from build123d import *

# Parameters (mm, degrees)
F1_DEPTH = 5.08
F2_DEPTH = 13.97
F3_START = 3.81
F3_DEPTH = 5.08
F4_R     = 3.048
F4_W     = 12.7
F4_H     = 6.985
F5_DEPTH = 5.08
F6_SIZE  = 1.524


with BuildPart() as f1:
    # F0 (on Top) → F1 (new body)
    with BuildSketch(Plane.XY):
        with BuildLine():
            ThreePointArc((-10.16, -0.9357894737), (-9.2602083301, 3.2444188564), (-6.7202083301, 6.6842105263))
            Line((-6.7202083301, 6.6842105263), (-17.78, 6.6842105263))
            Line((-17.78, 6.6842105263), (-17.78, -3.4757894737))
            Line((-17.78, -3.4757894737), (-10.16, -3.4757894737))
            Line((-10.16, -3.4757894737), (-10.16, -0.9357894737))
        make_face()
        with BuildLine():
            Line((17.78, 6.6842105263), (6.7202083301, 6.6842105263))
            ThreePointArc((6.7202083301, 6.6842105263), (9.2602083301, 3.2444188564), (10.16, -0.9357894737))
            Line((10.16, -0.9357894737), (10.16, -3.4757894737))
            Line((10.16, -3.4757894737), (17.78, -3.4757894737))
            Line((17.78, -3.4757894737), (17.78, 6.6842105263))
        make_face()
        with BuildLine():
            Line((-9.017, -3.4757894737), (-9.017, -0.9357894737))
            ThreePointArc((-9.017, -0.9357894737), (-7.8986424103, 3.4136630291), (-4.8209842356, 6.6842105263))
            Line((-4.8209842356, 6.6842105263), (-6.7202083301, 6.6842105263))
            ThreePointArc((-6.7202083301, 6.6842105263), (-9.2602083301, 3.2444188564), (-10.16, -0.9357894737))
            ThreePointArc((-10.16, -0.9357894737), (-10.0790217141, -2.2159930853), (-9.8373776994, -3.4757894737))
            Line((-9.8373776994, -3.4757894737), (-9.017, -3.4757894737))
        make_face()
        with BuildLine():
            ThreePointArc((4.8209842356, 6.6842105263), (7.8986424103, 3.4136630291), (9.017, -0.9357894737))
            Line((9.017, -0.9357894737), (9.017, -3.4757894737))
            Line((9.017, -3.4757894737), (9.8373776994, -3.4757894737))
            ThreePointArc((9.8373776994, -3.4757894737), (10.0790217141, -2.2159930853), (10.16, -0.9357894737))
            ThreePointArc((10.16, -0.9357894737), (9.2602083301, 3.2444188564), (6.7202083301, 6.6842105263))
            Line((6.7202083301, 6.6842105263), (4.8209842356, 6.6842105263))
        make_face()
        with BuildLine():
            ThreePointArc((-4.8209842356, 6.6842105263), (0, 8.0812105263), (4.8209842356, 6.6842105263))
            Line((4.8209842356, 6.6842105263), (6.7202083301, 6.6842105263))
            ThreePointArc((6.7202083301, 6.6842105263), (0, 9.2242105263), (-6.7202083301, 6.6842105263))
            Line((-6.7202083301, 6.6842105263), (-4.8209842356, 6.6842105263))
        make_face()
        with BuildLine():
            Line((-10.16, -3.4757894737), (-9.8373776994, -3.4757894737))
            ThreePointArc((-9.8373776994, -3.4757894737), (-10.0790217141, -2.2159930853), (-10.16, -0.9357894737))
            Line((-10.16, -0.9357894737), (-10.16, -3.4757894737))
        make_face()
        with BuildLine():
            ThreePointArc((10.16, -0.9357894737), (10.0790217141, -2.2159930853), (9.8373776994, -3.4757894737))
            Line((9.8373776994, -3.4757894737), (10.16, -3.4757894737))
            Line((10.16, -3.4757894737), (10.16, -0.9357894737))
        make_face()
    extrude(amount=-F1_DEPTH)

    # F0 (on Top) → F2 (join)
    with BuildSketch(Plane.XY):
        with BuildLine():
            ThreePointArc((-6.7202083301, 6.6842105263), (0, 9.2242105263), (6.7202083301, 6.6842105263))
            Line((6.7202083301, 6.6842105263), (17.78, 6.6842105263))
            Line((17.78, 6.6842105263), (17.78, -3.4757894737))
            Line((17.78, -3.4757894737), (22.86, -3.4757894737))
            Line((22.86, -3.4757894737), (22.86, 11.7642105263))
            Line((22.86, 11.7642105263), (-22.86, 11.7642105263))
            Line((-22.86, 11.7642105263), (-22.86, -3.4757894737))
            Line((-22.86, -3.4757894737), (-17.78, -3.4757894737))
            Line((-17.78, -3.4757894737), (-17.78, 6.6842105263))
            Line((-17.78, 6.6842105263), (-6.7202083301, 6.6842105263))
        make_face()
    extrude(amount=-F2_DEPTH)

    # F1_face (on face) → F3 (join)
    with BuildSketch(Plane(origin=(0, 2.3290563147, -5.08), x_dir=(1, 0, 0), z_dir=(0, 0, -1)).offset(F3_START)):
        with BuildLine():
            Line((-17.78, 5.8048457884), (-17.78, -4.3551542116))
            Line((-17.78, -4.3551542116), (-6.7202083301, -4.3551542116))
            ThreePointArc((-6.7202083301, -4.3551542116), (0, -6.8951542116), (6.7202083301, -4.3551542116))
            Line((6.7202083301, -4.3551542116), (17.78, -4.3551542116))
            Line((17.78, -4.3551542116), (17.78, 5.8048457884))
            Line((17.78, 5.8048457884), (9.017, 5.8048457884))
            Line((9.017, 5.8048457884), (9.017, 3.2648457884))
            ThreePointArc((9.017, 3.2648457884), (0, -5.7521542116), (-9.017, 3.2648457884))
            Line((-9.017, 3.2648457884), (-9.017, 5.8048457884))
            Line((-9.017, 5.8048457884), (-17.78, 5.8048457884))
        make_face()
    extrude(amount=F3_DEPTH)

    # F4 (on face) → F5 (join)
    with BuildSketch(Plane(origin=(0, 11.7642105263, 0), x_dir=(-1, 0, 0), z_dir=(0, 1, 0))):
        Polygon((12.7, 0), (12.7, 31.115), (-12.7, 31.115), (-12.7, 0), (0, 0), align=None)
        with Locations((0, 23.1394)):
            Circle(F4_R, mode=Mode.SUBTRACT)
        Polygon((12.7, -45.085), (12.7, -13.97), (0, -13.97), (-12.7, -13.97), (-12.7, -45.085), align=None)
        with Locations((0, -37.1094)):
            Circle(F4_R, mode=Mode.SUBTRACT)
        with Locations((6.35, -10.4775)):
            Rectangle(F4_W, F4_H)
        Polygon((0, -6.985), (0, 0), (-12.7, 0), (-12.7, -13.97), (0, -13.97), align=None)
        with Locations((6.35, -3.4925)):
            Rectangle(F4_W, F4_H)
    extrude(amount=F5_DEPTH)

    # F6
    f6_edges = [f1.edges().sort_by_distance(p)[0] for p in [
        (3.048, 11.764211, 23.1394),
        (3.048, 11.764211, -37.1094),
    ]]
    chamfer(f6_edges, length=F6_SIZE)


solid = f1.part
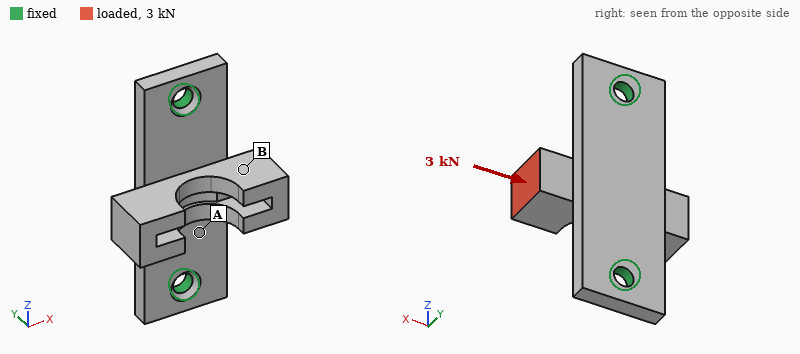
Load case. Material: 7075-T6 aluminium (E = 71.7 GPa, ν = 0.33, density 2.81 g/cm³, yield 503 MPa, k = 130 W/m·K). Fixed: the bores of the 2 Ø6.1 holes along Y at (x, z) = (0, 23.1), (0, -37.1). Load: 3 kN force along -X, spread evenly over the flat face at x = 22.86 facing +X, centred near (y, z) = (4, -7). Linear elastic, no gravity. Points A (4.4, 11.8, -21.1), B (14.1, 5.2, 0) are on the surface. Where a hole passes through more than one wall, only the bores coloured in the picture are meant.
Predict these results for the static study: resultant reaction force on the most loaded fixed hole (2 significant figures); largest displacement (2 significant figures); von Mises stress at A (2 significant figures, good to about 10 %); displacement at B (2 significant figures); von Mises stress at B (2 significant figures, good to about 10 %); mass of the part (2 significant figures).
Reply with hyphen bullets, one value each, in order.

- 1.5 kN
- 0.46 mm
- 140 MPa
- 0.26 mm
- 41 MPa
- 45 g
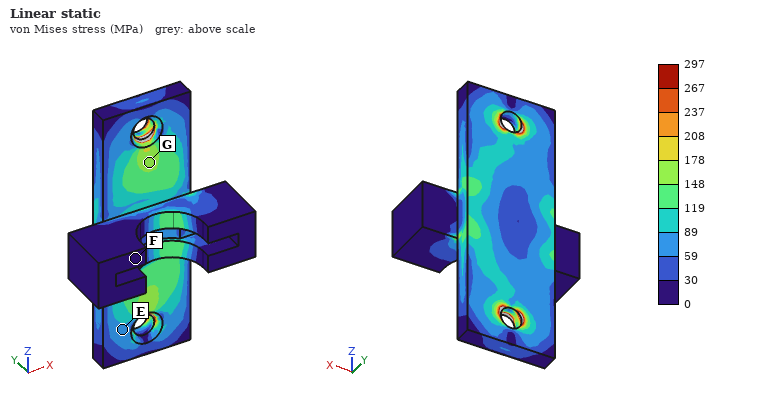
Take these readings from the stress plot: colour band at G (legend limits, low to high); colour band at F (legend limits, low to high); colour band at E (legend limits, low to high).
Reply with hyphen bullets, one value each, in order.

- 148 to 178 MPa
- 0 to 30 MPa
- 59 to 89 MPa
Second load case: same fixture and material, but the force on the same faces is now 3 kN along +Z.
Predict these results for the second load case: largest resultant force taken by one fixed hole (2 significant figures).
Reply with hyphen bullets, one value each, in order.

- 2.1 kN
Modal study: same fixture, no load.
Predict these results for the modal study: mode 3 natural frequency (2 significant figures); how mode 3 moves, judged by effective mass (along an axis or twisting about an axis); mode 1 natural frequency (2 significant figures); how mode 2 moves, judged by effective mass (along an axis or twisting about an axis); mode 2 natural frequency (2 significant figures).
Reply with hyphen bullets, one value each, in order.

- 8400 Hz
- along Z
- 3000 Hz
- along Y
- 4300 Hz
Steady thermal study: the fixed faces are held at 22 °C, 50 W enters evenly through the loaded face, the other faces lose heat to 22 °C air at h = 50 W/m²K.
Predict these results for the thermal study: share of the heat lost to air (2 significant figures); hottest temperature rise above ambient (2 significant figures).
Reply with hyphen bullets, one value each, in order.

- 19 %
- 84 K
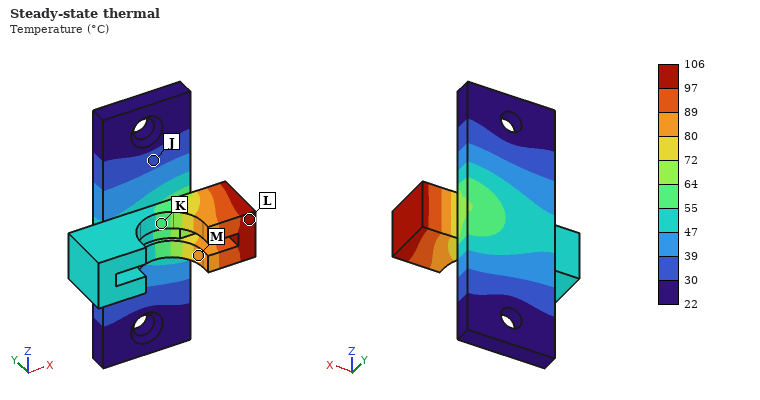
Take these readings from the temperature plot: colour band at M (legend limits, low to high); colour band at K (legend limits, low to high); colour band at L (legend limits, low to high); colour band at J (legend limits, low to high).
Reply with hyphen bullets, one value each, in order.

- 80 to 89 °C
- 55 to 64 °C
- 97 to 106 °C
- 30 to 39 °C
